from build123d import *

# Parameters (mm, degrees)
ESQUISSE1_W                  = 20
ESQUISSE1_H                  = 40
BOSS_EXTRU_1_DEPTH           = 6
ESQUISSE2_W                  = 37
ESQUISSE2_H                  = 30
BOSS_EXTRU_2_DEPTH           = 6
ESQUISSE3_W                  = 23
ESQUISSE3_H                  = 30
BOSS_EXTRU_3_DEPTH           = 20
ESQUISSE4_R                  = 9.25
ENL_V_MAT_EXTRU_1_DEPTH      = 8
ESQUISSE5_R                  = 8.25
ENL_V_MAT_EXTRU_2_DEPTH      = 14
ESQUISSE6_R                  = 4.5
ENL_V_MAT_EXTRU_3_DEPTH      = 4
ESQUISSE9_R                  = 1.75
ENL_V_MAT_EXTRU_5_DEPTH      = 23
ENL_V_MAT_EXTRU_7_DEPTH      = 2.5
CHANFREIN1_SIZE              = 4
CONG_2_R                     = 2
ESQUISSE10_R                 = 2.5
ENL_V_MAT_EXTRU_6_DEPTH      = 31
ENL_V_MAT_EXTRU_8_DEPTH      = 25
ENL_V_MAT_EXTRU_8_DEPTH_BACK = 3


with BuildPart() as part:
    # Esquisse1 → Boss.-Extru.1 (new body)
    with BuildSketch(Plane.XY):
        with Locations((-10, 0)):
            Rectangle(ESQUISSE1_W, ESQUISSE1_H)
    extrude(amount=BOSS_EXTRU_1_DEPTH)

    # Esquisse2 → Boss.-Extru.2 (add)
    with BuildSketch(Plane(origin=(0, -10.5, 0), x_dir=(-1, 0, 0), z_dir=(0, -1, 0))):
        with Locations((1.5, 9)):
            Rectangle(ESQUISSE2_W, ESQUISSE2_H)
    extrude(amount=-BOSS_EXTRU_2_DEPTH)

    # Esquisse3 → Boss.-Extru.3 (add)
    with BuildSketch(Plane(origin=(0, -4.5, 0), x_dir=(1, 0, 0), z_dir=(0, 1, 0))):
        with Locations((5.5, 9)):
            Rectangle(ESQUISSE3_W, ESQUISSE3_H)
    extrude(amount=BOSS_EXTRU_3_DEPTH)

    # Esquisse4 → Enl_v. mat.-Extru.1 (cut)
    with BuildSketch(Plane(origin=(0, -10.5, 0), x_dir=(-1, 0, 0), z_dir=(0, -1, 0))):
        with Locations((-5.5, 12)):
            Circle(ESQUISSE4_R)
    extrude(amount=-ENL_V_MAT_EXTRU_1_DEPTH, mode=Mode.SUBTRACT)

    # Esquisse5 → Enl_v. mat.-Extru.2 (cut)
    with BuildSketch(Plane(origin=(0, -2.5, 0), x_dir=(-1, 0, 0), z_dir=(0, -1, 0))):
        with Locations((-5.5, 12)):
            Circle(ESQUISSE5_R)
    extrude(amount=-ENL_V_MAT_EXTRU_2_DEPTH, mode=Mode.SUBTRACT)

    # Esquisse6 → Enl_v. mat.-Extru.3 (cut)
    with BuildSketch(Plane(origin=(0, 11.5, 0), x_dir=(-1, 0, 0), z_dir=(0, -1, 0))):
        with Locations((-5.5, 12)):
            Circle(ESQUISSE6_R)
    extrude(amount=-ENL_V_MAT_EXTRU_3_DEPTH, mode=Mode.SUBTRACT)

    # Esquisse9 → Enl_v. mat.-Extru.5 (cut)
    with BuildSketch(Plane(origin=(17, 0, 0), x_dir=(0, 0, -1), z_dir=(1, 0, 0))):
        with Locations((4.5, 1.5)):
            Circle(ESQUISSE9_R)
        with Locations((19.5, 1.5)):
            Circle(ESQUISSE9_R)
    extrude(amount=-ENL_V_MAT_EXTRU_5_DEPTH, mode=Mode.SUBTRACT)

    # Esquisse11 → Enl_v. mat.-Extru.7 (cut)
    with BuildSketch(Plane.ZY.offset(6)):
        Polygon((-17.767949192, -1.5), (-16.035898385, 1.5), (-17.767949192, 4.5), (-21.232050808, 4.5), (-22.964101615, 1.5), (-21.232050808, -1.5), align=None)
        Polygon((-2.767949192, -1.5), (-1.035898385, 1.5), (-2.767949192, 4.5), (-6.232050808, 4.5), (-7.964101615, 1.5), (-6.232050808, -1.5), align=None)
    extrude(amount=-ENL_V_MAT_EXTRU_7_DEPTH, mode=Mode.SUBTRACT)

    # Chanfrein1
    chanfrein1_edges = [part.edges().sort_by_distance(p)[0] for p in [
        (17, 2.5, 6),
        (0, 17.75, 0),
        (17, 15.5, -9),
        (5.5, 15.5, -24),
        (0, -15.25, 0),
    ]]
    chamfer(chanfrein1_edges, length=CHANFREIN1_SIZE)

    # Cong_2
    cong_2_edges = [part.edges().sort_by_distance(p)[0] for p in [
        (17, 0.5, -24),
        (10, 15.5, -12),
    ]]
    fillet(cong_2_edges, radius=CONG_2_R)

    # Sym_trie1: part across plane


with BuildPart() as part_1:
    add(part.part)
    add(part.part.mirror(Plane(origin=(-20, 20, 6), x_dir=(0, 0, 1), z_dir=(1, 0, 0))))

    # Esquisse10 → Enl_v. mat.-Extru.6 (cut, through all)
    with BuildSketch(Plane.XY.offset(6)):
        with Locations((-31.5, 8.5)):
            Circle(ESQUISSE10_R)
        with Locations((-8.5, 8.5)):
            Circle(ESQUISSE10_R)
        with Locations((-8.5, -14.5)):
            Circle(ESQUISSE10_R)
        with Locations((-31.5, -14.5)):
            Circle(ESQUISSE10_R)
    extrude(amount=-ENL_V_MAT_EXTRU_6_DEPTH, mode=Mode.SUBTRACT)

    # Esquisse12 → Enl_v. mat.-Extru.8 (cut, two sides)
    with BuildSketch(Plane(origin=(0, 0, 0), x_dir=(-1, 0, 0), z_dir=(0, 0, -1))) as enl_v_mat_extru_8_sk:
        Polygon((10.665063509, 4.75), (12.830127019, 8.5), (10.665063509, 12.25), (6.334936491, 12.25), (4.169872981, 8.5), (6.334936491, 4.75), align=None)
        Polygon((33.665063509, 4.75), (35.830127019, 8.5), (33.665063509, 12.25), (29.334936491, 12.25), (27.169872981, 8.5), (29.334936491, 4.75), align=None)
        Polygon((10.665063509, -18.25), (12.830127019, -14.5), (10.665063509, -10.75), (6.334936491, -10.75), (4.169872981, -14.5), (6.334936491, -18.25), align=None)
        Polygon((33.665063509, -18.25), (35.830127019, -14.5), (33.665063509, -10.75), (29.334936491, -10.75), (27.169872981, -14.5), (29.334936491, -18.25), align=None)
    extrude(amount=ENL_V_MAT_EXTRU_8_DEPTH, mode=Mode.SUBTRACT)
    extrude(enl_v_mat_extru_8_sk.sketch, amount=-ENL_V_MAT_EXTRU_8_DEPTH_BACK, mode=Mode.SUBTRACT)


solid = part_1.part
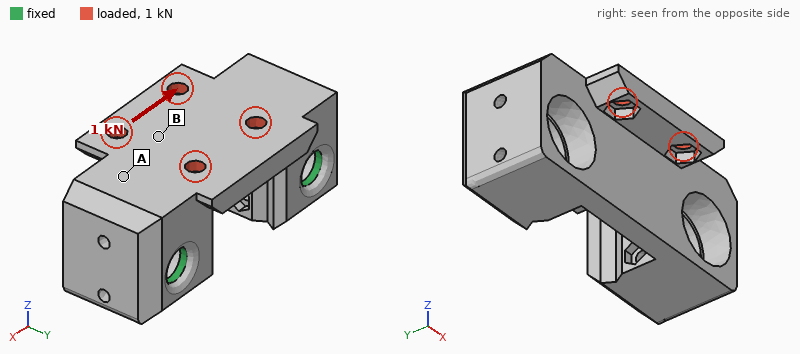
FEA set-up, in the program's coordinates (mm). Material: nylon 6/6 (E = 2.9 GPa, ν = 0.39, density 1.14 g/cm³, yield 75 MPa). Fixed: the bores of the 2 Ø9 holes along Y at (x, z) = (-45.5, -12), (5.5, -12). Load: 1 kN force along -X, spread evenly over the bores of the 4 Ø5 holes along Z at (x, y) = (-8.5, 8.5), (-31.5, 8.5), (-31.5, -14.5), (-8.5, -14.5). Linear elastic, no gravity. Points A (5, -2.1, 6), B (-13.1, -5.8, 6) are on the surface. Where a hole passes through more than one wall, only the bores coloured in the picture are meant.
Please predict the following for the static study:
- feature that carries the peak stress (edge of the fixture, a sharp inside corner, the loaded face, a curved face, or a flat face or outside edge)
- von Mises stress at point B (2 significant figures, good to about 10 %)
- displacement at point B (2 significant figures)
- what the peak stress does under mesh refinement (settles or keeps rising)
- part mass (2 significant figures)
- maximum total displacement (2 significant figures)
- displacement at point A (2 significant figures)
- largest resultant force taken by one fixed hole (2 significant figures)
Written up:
edge of the fixture
4.1 MPa
0.13 mm
keeps rising
38 g
0.18 mm
0.13 mm
620 N
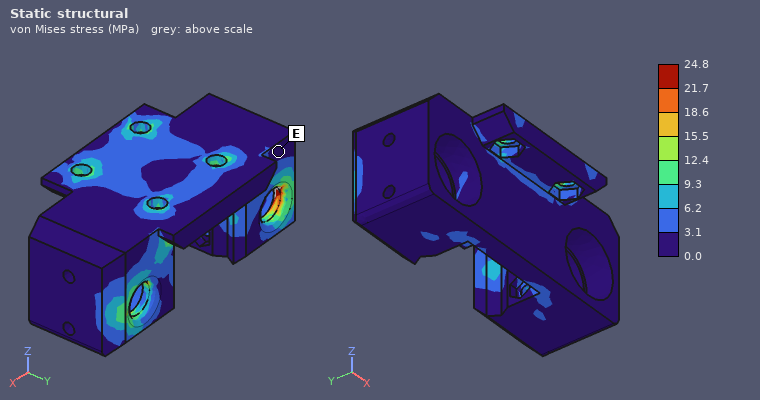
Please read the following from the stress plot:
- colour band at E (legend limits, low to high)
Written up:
0.0 to 3.1 MPa
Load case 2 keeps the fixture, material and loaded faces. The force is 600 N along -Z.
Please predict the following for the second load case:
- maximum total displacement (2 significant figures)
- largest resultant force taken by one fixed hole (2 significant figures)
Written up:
0.84 mm
330 N
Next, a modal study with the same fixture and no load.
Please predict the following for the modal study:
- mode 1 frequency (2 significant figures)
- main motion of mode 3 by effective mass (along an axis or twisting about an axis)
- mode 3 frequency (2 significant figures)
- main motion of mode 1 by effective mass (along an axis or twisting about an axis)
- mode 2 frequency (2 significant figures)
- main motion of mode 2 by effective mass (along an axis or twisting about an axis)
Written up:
970 Hz
along X
2800 Hz
along Z
2100 Hz
along X
